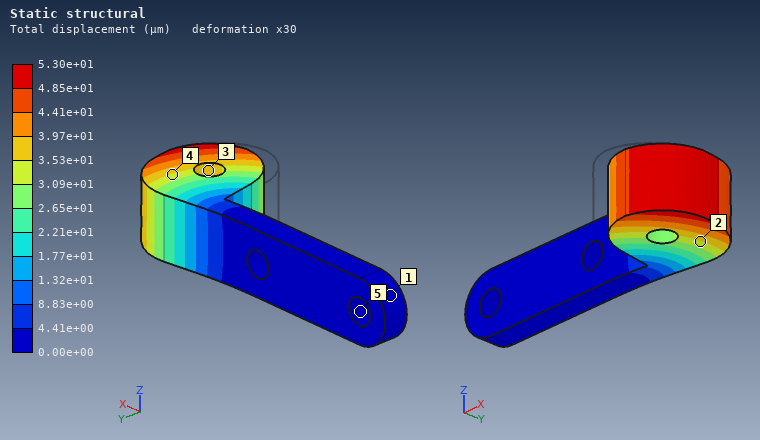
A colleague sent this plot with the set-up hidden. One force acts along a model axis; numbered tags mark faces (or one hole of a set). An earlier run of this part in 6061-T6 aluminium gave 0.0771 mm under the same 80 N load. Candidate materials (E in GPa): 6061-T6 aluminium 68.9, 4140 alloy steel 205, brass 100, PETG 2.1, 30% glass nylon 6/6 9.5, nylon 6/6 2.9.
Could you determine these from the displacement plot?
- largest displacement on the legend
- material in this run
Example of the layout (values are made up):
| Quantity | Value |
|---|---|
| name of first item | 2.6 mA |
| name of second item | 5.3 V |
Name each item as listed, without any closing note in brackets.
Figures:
| Quantity | Value |
|---|---|
| largest displacement on the legend | 5.30e+01 µm |
| material in this run | brass |
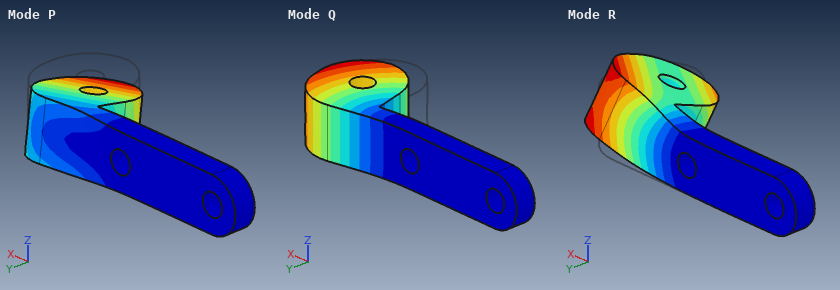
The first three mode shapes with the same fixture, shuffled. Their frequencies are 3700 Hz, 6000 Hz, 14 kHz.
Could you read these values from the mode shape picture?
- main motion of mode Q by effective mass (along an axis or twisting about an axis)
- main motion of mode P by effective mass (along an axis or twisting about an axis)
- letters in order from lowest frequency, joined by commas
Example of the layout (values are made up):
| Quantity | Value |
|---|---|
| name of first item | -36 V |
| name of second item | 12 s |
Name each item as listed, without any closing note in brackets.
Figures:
| Quantity | Value |
|---|---|
| main motion of mode Q by effective mass | along Y |
| main motion of mode P by effective mass | along Z |
| letters in order from lowest frequency, joined by commas | Q, P, R |
